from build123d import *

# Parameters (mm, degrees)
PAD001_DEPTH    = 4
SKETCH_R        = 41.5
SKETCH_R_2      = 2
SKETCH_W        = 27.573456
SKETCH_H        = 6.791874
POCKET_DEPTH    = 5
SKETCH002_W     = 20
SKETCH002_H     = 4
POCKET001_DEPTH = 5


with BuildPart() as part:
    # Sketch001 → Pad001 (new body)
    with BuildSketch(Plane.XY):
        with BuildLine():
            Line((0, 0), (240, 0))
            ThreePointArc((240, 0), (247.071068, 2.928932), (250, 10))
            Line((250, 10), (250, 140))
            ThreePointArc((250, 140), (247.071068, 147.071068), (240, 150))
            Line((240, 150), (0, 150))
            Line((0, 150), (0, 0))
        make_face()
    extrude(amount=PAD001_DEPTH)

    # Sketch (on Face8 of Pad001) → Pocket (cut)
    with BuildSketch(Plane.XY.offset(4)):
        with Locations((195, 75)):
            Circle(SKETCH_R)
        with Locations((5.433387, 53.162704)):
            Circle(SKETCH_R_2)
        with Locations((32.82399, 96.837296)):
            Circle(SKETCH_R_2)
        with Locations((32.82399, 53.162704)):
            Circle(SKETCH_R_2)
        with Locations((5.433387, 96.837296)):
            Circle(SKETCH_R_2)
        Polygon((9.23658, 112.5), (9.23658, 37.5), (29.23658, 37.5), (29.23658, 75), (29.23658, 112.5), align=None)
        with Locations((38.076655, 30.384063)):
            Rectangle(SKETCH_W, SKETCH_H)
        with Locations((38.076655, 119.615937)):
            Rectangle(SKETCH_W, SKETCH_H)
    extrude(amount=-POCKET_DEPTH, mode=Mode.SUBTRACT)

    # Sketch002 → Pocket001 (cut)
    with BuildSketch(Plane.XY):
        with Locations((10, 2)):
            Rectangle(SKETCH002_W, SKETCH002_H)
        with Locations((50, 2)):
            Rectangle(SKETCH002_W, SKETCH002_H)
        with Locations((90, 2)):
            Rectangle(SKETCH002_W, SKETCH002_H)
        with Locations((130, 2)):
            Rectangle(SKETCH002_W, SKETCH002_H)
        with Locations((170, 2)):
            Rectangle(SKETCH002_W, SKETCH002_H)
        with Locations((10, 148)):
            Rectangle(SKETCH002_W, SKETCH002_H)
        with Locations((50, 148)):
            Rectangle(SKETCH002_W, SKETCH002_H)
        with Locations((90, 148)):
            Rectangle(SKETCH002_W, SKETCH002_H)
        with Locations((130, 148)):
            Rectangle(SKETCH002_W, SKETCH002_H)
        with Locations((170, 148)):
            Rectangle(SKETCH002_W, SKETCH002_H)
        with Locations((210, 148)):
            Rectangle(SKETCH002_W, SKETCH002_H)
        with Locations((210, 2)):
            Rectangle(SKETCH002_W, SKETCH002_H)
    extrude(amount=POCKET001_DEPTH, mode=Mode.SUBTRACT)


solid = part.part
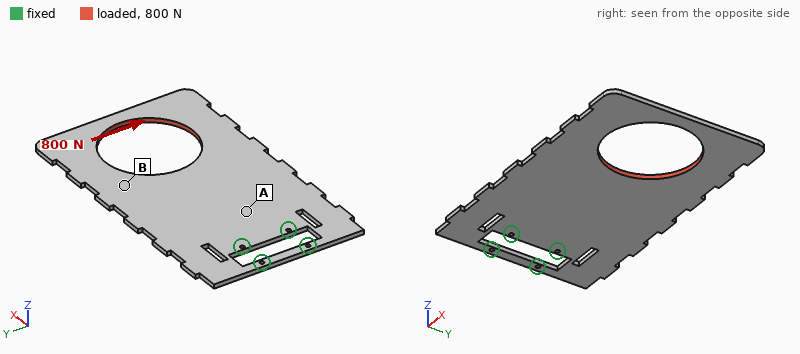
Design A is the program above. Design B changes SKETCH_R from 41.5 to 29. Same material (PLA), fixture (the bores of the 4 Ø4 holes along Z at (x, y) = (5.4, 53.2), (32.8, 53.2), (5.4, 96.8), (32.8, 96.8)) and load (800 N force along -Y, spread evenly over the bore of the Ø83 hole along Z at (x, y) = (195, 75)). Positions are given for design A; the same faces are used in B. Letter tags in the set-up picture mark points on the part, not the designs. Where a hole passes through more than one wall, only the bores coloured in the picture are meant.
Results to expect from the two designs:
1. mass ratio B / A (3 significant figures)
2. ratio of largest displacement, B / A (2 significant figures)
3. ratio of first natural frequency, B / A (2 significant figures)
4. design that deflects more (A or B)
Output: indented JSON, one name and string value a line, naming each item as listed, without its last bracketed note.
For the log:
{
  "mass ratio B / A": "1.09",
  "ratio of largest displacement, B / A": "0.90",
  "ratio of first natural frequency, B / A": "0.91",
  "design that deflects more": "A"
}
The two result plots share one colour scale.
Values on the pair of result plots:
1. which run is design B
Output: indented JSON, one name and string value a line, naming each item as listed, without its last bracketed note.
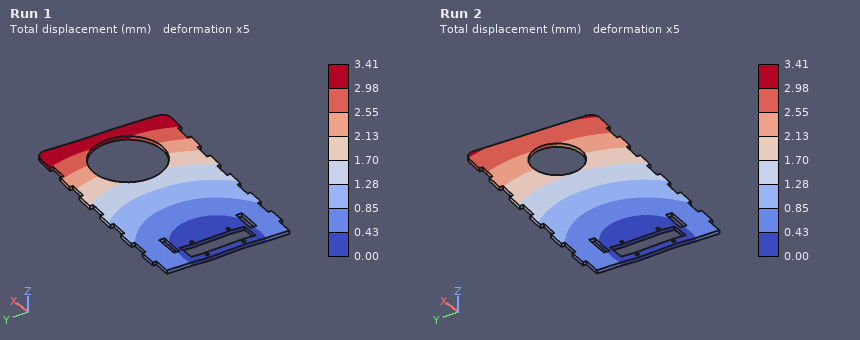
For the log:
{
  "which run is design B": "Run 2"
}
